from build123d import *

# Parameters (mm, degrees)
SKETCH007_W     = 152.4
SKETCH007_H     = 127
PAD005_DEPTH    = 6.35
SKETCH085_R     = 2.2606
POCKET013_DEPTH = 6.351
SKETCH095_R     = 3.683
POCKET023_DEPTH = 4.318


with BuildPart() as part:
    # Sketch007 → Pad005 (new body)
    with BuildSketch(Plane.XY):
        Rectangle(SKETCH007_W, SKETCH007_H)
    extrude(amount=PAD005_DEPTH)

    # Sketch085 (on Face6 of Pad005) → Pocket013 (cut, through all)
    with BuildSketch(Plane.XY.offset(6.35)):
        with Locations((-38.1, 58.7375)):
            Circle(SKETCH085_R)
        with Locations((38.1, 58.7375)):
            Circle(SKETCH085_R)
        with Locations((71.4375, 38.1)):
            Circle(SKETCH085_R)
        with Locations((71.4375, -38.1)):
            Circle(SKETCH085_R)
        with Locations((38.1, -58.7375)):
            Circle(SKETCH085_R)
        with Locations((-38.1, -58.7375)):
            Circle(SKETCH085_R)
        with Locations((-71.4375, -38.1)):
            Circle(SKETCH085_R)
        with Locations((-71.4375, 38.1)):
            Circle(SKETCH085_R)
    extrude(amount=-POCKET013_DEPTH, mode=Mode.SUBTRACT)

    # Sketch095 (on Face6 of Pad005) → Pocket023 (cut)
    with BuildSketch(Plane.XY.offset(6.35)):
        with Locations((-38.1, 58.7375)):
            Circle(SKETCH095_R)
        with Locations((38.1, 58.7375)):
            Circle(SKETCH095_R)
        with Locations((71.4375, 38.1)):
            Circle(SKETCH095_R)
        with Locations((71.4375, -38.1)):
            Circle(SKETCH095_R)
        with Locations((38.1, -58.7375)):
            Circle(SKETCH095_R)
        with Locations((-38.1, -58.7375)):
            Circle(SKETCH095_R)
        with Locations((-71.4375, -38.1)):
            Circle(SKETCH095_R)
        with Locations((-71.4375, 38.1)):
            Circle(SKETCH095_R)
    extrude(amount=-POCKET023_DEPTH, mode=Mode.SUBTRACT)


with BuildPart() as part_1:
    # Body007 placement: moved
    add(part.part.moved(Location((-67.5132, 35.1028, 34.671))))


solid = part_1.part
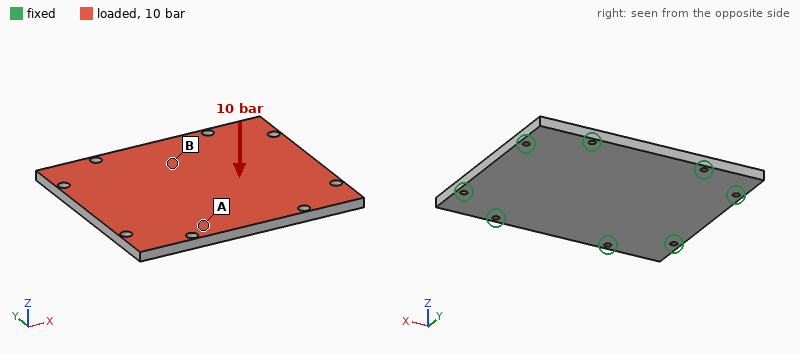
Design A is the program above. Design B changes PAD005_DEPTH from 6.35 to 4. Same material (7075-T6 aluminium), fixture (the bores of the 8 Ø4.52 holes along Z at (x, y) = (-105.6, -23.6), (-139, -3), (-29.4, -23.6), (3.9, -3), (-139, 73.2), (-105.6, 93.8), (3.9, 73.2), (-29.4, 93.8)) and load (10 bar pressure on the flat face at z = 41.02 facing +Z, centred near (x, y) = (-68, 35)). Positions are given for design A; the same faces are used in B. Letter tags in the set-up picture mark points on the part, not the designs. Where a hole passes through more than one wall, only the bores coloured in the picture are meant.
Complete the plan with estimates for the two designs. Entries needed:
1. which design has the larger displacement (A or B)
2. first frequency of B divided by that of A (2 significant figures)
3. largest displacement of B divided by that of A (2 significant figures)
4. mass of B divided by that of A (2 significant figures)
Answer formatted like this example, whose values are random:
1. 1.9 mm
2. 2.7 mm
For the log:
1. B
2. 0.70
3. 3.3
4. 0.63
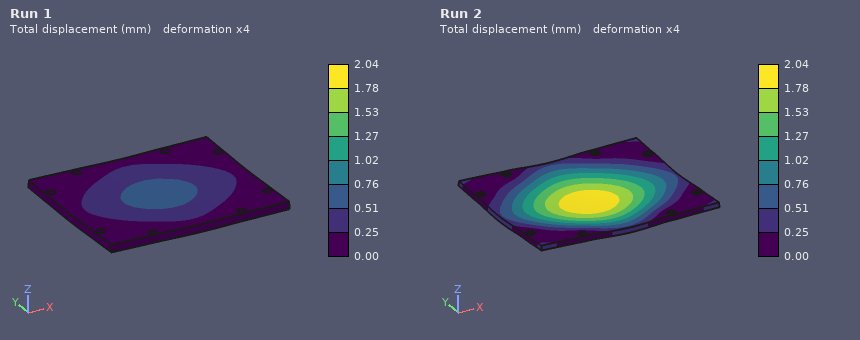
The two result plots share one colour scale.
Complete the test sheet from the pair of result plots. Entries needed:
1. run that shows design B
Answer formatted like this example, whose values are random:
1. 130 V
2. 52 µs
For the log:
1. Run 2
